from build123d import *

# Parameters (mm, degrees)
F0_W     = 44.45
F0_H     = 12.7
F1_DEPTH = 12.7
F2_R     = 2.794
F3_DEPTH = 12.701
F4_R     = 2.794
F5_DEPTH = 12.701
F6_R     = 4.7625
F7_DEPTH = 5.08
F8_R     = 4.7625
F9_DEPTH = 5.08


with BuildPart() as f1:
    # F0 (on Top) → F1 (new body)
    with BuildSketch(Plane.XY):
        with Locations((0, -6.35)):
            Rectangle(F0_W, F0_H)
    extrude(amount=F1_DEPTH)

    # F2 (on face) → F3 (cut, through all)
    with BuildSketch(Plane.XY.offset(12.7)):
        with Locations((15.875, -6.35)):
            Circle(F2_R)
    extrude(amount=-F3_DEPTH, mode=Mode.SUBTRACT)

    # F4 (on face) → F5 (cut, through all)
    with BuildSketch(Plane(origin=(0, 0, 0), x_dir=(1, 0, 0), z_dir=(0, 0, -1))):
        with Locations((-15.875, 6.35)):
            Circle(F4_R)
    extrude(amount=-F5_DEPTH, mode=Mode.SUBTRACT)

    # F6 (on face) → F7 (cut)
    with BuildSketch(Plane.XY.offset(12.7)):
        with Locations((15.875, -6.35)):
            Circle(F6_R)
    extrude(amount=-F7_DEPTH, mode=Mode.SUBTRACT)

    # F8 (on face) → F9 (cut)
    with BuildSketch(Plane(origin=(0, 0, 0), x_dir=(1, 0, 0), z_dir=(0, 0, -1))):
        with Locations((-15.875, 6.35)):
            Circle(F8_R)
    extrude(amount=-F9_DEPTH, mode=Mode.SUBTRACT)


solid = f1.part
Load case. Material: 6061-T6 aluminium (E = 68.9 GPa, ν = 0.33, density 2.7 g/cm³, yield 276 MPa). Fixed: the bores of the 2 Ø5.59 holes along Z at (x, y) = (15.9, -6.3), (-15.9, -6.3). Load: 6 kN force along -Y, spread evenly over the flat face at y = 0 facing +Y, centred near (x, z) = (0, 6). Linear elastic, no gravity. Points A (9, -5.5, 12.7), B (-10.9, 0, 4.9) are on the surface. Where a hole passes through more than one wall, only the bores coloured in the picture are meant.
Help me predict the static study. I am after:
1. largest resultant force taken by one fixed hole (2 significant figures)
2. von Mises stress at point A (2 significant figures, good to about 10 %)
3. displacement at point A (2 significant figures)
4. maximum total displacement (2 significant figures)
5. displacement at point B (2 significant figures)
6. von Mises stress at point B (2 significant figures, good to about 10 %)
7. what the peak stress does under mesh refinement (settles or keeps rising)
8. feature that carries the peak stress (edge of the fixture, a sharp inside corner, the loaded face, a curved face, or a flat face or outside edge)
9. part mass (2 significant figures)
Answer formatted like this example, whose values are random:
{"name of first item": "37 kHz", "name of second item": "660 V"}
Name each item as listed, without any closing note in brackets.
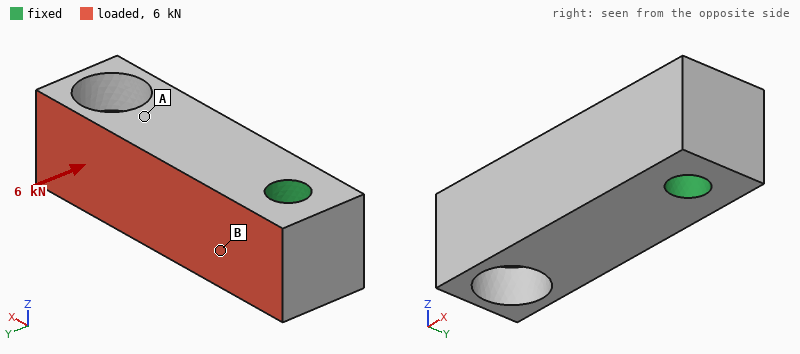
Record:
{"largest resultant force taken by one fixed hole": "3.0 kN", "von Mises stress at point A": "13 MPa", "displacement at point A": "8.3 µm", "maximum total displacement": "13 µm", "displacement at point B": "6.6 µm", "von Mises stress at point B": "31 MPa", "what the peak stress does under mesh refinement": "keeps rising", "feature that carries the peak stress": "edge of the fixture", "part mass": "16 g"}
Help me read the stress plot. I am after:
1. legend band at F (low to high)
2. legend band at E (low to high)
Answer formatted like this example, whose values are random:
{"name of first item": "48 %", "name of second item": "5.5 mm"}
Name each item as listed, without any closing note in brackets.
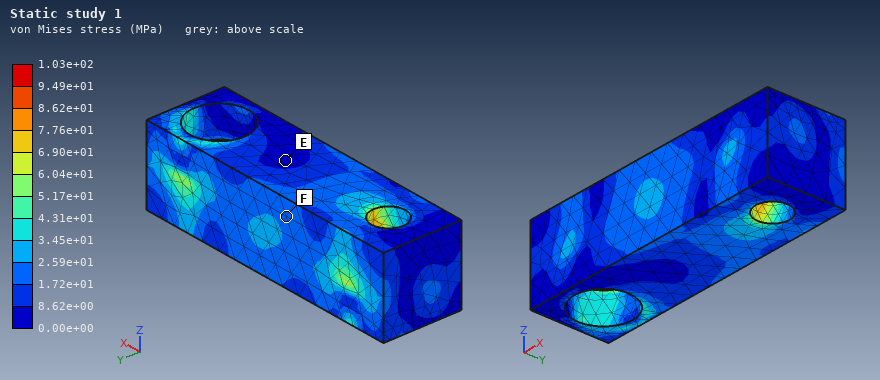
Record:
{"legend band at F": "1.72e+01 to 2.59e+01 MPa", "legend band at E": "0.00e+00 to 8.62e+00 MPa"}
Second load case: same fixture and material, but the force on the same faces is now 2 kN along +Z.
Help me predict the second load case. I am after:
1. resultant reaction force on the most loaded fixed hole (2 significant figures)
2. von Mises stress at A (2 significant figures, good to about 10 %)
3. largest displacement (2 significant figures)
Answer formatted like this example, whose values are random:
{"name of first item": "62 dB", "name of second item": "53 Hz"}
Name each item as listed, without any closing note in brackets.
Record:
{"resultant reaction force on the most loaded fixed hole": "1.0 kN", "von Mises stress at A": "12 MPa", "largest displacement": "8.7 µm"}
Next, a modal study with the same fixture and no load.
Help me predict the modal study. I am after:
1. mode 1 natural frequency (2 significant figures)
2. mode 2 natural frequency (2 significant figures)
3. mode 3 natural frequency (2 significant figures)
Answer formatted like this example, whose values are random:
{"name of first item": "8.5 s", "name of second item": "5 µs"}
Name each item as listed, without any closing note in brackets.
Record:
{"mode 1 natural frequency": "32 kHz", "mode 2 natural frequency": "33 kHz", "mode 3 natural frequency": "34 kHz"}
